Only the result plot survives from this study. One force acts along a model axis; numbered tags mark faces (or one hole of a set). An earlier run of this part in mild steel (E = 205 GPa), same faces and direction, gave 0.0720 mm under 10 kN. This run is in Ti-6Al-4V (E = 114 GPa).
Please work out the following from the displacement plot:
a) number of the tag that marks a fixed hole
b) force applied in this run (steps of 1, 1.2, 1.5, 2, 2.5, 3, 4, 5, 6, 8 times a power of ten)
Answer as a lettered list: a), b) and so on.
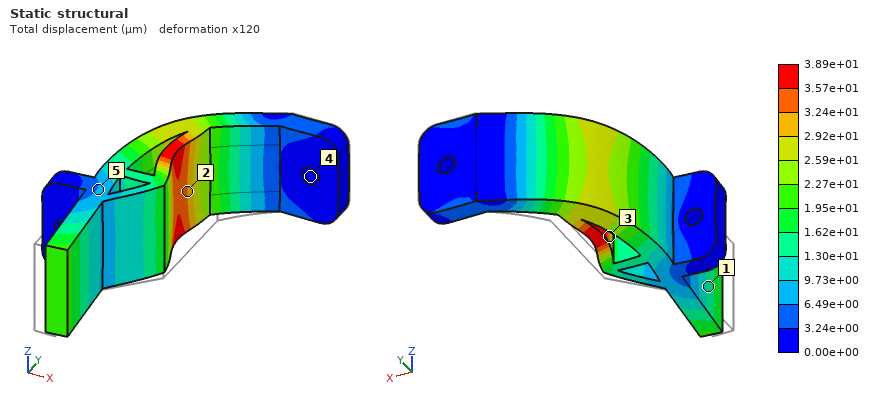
a) 4
b) 3 kN
